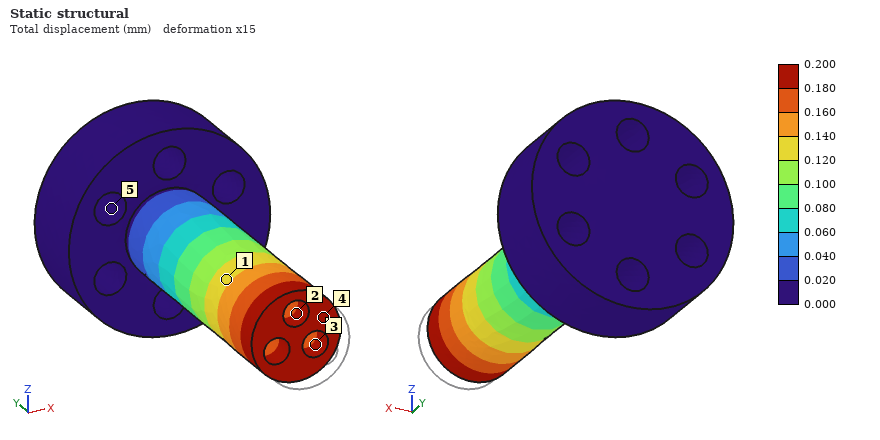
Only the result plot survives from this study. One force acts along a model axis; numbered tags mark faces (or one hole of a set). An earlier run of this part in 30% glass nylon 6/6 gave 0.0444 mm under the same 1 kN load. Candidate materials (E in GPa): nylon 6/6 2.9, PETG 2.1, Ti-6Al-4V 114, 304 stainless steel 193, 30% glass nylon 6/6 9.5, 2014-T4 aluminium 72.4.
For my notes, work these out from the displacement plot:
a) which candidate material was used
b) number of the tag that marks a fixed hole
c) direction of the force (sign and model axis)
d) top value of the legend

PETG
5
+Y
0.200 mm
